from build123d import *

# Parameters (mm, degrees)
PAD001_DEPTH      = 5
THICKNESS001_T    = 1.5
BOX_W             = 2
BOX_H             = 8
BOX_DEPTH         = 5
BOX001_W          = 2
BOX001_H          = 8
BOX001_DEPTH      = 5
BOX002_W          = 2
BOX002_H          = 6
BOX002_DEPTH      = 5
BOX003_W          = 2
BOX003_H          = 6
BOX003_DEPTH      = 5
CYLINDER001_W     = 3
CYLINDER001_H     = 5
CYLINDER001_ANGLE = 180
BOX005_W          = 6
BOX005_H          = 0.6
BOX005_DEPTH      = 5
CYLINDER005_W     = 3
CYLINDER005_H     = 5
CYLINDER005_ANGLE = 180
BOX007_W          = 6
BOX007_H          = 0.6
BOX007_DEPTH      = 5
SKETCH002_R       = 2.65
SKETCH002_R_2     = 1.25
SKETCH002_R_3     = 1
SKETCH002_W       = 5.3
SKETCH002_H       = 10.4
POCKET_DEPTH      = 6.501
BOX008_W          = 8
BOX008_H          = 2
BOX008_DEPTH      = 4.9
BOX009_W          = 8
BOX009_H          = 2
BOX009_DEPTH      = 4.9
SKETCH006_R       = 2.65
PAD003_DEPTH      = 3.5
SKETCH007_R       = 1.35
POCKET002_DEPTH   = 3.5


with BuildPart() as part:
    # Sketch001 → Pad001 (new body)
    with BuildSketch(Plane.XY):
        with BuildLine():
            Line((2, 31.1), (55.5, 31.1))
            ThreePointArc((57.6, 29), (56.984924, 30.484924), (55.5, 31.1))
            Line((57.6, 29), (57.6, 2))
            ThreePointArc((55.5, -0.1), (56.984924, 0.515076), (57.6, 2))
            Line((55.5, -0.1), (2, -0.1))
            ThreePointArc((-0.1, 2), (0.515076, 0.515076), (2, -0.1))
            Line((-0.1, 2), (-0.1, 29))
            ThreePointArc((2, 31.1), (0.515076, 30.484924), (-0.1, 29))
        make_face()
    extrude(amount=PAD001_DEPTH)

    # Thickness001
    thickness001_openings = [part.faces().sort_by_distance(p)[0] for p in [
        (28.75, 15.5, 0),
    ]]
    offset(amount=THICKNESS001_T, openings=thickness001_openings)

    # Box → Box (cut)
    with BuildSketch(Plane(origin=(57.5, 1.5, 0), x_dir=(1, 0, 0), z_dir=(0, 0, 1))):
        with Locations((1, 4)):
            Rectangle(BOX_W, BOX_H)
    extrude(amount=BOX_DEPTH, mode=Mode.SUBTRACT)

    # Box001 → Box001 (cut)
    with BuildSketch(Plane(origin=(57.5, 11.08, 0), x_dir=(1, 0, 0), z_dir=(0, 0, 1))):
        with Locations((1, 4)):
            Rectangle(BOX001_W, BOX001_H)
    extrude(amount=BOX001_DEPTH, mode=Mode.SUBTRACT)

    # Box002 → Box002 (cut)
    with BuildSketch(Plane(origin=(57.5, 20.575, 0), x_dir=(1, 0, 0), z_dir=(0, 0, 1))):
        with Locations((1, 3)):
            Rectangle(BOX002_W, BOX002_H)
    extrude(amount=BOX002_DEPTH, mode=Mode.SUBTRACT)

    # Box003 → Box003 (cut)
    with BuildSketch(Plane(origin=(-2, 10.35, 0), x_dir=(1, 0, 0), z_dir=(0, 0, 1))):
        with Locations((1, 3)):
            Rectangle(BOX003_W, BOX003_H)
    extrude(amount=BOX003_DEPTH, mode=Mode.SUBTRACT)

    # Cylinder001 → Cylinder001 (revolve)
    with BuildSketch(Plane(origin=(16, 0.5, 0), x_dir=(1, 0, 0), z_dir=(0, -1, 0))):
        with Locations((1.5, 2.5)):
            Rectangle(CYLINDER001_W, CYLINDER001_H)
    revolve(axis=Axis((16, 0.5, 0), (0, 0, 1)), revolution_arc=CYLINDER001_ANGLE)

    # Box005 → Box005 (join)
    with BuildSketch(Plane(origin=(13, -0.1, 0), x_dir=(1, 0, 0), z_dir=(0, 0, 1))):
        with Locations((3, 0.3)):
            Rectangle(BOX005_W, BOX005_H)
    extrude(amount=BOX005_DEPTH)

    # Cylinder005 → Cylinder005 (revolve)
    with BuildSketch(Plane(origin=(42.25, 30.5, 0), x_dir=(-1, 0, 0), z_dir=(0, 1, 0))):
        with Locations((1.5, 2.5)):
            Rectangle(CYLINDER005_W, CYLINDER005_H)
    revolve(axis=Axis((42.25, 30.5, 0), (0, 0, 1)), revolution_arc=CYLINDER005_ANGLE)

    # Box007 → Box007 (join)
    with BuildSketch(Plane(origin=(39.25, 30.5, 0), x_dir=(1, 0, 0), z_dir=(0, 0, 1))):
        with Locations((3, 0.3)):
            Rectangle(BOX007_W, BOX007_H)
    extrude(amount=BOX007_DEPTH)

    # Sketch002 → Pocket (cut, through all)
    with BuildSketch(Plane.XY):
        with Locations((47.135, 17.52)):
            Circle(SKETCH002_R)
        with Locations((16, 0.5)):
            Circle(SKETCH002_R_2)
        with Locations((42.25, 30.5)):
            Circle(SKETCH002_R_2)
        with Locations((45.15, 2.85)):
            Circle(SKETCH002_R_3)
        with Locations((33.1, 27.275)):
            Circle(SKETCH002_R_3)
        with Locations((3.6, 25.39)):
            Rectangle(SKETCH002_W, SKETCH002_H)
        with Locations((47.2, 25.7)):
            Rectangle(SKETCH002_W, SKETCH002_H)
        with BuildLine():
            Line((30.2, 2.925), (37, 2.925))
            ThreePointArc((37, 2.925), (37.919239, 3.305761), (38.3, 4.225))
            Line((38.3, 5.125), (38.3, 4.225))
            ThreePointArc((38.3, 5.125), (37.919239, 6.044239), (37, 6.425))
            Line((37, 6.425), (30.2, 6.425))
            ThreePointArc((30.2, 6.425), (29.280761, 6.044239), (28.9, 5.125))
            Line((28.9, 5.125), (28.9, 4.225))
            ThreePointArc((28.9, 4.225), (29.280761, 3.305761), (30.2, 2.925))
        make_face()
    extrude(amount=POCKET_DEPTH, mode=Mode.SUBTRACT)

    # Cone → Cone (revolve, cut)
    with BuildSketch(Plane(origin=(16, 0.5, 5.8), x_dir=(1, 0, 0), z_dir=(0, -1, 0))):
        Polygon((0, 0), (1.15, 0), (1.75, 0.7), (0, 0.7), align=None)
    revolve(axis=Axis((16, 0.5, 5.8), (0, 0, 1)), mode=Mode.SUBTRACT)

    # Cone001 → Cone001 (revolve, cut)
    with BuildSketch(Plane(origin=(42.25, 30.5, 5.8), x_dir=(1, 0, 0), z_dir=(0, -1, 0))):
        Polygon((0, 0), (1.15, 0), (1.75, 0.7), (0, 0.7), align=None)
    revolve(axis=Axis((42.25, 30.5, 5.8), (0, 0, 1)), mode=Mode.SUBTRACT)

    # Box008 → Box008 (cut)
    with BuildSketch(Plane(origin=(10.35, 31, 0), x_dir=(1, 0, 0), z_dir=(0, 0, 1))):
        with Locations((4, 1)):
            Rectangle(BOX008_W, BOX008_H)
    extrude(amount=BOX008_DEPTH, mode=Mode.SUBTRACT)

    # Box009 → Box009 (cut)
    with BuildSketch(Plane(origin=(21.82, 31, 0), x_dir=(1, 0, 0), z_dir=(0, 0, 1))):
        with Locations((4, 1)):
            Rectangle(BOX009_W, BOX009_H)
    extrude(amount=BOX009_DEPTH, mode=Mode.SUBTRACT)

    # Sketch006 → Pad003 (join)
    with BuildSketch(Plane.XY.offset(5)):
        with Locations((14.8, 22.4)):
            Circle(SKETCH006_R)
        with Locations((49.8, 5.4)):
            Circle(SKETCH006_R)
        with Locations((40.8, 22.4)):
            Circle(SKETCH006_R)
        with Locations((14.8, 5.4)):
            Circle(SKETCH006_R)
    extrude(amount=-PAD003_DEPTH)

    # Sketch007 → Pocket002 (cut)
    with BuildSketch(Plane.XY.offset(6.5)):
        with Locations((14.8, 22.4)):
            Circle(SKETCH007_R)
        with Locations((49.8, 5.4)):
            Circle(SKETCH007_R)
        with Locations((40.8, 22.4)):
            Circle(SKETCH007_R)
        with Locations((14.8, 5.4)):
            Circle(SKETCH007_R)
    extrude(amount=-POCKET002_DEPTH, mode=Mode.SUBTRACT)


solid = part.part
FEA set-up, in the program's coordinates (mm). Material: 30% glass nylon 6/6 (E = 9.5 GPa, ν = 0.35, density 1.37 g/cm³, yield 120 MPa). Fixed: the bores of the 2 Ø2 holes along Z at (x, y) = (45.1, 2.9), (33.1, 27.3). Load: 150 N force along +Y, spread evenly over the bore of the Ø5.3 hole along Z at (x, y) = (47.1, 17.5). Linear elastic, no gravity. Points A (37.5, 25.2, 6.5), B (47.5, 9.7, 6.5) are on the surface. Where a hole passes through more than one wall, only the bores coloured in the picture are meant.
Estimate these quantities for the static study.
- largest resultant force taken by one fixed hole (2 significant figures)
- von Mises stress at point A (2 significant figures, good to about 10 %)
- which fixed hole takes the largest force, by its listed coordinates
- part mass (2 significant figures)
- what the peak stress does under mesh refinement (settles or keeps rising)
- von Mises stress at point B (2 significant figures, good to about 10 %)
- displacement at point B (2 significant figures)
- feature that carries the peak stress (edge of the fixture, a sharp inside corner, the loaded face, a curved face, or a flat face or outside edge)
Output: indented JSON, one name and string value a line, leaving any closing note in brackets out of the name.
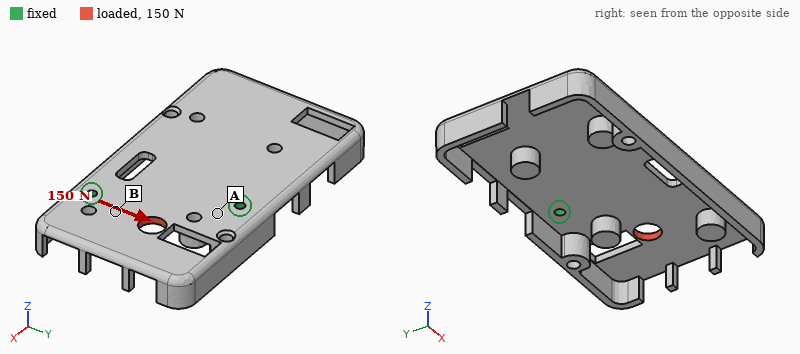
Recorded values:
{
  "largest resultant force taken by one fixed hole": "110 N",
  "von Mises stress at point A": "3.4 MPa",
  "which fixed hole takes the largest force, by its listed coordinates": "(45.1, 2.9)",
  "part mass": "5.6 g",
  "what the peak stress does under mesh refinement": "keeps rising",
  "von Mises stress at point B": "8.4 MPa",
  "displacement at point B": "8.0 µm",
  "feature that carries the peak stress": "a sharp inside corner"
}
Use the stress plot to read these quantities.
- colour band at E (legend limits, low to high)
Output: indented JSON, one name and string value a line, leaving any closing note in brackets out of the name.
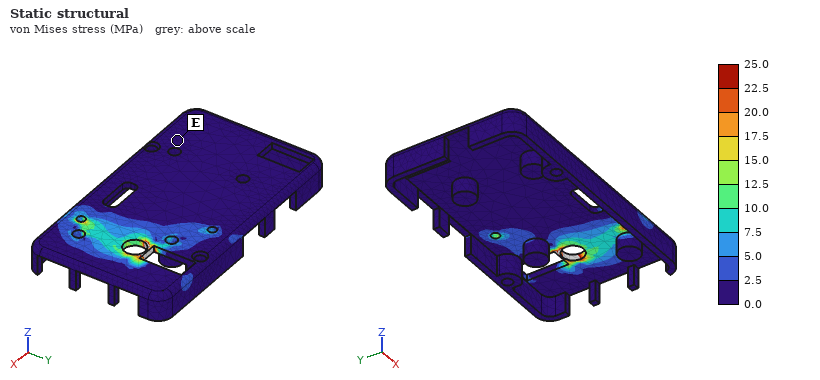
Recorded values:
{
  "colour band at E": "0.0 to 2.5 MPa"
}
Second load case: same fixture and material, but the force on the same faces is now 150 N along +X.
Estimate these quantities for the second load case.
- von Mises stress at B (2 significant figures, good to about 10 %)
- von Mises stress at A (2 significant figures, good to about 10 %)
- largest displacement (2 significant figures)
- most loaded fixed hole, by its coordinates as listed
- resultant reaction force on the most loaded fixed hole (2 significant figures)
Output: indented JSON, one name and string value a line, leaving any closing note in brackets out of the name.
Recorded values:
{
  "von Mises stress at B": "1.8 MPa",
  "von Mises stress at A": "4.4 MPa",
  "largest displacement": "53 µm",
  "most loaded fixed hole, by its coordinates as listed": "(33.1, 27.3)",
  "resultant reaction force on the most loaded fixed hole": "87 N"
}
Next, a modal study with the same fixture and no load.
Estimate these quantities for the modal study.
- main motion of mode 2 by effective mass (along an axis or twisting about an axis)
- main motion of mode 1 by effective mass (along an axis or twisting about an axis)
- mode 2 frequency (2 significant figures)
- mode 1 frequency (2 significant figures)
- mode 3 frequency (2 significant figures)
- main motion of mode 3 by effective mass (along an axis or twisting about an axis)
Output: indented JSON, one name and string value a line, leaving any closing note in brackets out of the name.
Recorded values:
{
  "main motion of mode 2 by effective mass": "twisting about X",
  "main motion of mode 1 by effective mass": "along Z",
  "mode 2 frequency": "1000 Hz",
  "mode 1 frequency": "500 Hz",
  "mode 3 frequency": "1500 Hz",
  "main motion of mode 3 by effective mass": "along Z"
}
